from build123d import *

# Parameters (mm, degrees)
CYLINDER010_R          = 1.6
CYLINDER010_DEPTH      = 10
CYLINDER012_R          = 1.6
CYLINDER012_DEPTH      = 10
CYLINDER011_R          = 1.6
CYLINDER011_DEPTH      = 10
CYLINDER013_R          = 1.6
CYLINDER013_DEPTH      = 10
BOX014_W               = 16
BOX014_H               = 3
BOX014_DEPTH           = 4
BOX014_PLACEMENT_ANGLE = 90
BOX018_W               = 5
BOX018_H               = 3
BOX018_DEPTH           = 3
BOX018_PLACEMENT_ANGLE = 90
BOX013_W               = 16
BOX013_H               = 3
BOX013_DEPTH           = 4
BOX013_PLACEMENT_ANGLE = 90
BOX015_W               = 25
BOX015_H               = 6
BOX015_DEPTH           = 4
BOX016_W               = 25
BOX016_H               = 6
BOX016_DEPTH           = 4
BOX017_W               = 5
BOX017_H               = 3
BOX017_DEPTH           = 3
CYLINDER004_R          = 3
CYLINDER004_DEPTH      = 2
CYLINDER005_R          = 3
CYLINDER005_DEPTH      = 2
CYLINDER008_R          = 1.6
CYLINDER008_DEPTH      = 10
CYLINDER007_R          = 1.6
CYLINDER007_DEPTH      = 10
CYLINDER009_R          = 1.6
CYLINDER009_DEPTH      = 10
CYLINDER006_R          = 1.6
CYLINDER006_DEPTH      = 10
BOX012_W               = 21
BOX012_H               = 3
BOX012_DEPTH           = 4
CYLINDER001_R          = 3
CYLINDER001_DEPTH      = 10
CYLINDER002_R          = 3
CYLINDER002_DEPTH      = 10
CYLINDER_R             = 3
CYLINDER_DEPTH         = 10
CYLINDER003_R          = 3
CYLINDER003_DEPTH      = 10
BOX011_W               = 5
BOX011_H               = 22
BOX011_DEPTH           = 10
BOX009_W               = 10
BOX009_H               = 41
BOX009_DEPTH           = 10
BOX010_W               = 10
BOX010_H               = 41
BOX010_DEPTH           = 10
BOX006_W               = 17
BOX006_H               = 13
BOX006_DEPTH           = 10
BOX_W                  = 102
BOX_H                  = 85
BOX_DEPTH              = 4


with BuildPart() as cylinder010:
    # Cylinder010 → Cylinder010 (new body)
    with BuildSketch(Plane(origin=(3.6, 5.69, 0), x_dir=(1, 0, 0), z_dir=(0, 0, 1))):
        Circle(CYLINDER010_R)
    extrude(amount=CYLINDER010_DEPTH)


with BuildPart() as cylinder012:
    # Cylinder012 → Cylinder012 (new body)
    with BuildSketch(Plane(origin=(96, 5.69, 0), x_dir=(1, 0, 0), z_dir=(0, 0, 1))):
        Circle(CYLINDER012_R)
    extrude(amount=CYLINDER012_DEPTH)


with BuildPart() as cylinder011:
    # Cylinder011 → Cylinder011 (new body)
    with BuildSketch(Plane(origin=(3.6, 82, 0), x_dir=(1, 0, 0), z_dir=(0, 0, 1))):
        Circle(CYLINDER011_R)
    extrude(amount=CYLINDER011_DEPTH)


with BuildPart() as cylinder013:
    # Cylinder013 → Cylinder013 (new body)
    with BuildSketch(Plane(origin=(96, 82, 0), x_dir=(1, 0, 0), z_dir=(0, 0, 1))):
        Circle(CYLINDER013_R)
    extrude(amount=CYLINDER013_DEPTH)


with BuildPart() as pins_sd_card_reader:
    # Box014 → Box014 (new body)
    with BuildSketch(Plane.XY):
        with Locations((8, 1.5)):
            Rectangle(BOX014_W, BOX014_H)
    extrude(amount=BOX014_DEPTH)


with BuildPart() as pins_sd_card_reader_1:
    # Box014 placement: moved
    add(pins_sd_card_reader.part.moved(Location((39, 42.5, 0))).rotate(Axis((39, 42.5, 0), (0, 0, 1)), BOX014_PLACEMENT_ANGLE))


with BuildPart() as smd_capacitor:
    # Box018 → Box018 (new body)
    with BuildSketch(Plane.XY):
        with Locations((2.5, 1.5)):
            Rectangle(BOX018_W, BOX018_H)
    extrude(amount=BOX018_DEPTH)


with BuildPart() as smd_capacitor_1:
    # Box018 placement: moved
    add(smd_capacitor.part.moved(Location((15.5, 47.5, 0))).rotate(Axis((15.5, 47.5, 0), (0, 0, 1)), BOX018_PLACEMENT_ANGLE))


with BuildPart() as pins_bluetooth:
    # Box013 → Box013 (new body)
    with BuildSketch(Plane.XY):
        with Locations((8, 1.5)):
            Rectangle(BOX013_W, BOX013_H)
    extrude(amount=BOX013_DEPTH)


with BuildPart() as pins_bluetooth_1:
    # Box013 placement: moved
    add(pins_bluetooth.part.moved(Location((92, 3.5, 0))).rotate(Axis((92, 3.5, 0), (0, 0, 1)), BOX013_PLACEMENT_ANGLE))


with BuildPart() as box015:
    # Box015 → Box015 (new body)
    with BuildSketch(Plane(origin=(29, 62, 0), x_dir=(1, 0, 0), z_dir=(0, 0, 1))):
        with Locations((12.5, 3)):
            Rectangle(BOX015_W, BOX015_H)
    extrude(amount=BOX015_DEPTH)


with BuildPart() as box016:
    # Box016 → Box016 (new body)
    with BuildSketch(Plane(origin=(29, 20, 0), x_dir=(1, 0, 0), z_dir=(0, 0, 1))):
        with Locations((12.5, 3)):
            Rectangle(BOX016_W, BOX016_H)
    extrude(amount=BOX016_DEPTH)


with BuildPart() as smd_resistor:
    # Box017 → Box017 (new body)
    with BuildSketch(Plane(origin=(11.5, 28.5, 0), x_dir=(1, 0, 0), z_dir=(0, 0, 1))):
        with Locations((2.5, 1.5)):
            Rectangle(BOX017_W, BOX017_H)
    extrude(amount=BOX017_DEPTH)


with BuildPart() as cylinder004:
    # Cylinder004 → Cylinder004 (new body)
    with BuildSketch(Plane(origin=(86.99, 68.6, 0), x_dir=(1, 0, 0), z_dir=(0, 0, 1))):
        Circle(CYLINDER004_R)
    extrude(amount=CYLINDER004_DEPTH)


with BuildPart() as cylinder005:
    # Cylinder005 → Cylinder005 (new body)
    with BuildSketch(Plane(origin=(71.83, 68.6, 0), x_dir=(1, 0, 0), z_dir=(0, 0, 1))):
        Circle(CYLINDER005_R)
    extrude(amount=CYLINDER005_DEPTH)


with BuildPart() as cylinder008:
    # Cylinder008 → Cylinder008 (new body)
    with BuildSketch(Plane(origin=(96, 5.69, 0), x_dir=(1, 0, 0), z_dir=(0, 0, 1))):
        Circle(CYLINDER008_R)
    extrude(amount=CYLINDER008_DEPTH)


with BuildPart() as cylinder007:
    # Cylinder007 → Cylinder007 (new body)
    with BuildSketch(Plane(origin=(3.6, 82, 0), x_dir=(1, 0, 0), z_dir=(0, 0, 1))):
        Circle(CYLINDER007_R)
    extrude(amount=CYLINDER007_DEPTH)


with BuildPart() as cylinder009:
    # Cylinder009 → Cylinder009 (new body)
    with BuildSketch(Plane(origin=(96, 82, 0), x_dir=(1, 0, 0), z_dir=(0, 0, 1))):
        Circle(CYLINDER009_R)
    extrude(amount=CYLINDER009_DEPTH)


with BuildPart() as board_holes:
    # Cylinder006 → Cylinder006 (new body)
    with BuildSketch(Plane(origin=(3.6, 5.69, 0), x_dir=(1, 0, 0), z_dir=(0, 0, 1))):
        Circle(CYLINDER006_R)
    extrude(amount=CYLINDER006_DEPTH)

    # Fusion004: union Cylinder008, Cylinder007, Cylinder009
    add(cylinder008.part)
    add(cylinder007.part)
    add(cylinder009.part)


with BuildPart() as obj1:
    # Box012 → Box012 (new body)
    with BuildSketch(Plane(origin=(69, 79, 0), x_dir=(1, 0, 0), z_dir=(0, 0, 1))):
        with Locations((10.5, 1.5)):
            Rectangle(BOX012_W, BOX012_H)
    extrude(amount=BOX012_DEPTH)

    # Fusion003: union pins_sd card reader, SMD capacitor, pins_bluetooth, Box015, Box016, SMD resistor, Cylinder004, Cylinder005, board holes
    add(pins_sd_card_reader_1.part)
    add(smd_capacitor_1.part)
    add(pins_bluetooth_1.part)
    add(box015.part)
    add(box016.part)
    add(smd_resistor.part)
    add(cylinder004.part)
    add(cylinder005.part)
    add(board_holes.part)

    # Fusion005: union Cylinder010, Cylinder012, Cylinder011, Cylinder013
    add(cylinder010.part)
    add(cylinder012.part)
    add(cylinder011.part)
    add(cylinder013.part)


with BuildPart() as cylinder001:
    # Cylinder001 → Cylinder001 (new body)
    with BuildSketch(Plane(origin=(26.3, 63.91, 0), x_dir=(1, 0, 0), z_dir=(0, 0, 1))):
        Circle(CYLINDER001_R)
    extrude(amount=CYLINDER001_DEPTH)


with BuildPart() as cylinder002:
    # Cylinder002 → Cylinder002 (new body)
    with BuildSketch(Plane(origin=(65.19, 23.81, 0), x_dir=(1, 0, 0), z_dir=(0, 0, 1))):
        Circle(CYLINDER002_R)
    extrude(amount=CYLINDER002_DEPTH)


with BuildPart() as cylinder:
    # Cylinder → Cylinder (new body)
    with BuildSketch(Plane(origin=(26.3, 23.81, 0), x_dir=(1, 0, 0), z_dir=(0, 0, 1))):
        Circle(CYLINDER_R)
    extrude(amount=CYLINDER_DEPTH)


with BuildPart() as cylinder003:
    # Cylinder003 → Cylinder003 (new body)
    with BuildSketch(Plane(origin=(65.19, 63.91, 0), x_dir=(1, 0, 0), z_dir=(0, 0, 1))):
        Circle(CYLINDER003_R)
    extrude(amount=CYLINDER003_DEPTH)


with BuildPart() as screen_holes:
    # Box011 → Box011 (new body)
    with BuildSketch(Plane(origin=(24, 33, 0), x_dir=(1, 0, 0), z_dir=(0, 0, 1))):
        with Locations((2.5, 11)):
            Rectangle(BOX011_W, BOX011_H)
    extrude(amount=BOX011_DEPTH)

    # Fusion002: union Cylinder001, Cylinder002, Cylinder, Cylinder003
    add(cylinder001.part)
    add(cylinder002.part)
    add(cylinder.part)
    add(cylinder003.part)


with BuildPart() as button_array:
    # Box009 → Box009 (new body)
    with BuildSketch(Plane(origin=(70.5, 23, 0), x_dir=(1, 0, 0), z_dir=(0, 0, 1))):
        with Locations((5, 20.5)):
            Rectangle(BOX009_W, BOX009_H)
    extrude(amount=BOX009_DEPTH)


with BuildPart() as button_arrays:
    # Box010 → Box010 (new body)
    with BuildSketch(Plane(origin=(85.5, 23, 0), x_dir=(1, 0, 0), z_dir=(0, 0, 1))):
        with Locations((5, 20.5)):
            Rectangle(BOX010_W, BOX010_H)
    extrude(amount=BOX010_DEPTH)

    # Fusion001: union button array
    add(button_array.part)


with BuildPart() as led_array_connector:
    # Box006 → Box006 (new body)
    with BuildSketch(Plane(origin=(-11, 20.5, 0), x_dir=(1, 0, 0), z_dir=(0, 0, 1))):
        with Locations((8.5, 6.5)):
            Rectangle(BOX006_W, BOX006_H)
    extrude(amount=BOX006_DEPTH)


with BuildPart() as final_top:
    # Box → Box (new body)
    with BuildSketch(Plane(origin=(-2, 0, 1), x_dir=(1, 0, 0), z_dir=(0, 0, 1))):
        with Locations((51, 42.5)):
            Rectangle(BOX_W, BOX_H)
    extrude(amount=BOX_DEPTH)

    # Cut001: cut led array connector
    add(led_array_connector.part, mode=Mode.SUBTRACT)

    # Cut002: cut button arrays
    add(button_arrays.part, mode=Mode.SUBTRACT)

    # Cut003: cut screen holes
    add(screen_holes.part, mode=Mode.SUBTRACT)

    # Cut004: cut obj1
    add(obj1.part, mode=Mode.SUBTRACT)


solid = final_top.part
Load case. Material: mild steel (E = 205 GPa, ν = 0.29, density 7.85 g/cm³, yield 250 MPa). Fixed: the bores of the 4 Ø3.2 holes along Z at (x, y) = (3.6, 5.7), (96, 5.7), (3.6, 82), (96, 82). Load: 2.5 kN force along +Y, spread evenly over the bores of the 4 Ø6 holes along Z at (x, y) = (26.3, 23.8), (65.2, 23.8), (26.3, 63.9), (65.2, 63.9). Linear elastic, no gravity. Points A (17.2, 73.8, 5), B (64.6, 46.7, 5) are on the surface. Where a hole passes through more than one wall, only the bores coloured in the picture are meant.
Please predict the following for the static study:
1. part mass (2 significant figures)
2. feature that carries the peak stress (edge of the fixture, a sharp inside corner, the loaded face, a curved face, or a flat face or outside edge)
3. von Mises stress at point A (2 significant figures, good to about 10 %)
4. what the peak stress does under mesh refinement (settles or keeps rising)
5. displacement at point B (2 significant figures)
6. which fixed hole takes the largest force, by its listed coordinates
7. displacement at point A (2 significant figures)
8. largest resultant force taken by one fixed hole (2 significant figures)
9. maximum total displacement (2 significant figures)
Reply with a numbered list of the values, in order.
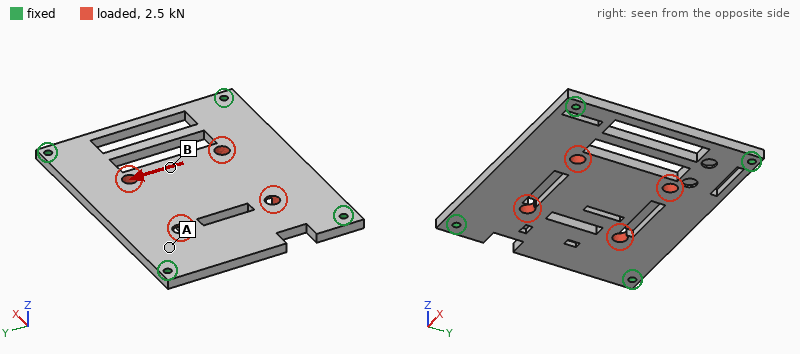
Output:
1. 220 g
2. edge of the fixture
3. 13 MPa
4. keeps rising
5. 6.6 µm
6. (3.6, 82)
7. 2.5 µm
8. 1.3 kN
9. 7.2 µm
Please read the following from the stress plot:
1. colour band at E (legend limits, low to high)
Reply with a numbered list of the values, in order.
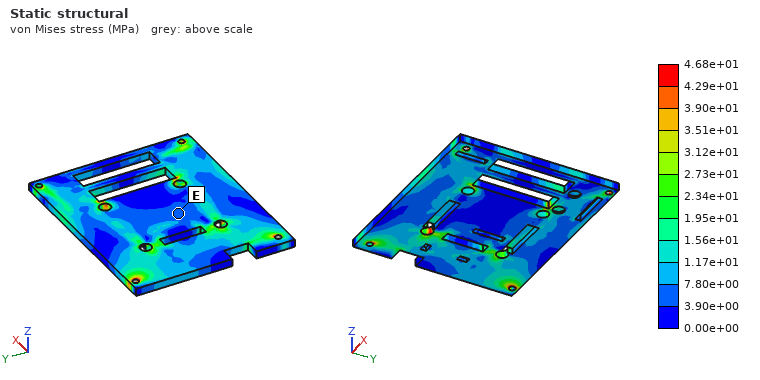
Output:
1. 3.90e+00 to 7.80e+00 MPa
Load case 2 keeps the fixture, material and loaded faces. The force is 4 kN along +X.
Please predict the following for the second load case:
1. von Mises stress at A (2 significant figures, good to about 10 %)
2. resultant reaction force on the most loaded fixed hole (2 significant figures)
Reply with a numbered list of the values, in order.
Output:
1. 16 MPa
2. 1.3 kN
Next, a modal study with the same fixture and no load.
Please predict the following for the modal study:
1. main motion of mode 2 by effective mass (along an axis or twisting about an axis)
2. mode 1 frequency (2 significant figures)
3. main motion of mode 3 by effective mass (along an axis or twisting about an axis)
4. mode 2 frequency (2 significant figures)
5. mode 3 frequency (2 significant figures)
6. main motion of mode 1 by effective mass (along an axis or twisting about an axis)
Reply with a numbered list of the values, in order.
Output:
1. twisting about X
2. 1600 Hz
3. twisting about Y
4. 2600 Hz
5. 3300 Hz
6. along Z
